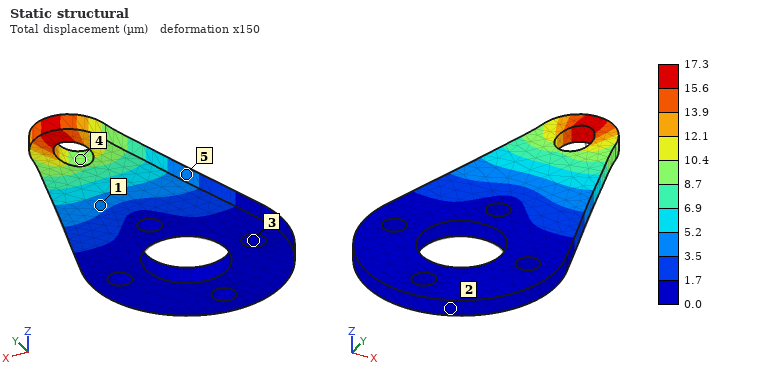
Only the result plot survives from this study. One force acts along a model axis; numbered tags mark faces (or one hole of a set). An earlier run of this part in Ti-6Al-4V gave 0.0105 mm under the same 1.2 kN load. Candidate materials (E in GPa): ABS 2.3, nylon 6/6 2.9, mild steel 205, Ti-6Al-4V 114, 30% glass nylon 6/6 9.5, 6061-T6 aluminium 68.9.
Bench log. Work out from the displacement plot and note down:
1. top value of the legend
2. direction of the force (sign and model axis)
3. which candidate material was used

17.3 µm
+Y
6061-T6 aluminium
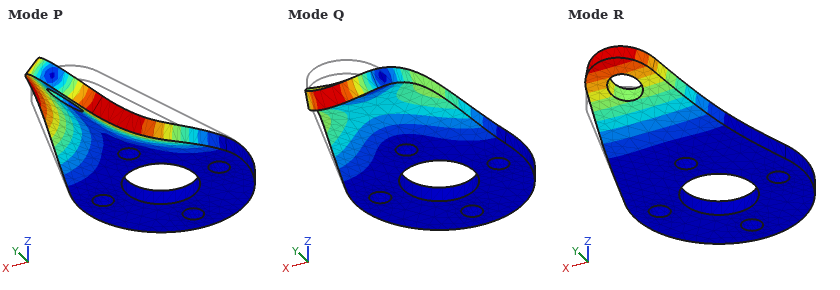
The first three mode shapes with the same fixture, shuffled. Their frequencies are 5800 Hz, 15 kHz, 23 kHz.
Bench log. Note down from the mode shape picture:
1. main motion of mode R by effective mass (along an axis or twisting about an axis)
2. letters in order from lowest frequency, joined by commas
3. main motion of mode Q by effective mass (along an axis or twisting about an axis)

along Z
R, P, Q
along Z
